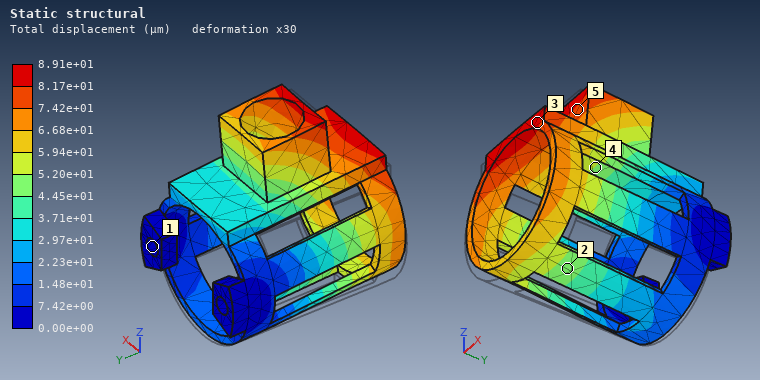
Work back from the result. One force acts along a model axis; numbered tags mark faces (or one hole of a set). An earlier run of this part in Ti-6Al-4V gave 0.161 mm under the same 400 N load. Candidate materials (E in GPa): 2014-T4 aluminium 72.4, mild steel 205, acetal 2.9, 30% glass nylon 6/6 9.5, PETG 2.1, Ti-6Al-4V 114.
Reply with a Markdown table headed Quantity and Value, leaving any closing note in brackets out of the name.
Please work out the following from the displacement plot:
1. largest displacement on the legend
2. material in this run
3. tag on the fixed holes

| Quantity | Value |
|---|---|
| largest displacement on the legend | 8.91e+01 µm |
| material in this run | mild steel |
| tag on the fixed holes | 1 |
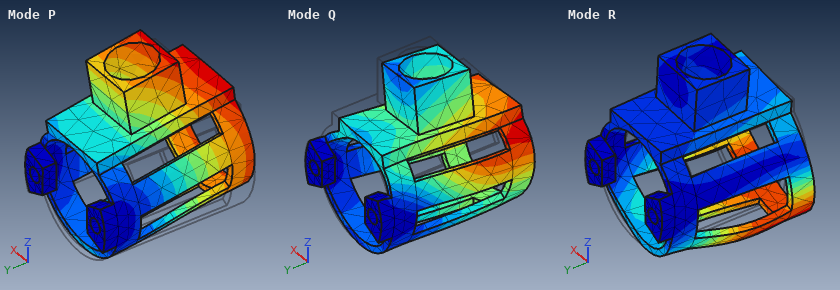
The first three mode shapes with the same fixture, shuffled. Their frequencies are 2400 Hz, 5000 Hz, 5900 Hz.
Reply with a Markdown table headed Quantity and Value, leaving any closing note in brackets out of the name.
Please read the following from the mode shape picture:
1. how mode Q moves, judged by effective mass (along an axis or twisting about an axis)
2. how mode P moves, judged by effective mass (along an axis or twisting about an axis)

| Quantity | Value |
|---|---|
| how mode Q moves, judged by effective mass | along X |
| how mode P moves, judged by effective mass | along Z |
